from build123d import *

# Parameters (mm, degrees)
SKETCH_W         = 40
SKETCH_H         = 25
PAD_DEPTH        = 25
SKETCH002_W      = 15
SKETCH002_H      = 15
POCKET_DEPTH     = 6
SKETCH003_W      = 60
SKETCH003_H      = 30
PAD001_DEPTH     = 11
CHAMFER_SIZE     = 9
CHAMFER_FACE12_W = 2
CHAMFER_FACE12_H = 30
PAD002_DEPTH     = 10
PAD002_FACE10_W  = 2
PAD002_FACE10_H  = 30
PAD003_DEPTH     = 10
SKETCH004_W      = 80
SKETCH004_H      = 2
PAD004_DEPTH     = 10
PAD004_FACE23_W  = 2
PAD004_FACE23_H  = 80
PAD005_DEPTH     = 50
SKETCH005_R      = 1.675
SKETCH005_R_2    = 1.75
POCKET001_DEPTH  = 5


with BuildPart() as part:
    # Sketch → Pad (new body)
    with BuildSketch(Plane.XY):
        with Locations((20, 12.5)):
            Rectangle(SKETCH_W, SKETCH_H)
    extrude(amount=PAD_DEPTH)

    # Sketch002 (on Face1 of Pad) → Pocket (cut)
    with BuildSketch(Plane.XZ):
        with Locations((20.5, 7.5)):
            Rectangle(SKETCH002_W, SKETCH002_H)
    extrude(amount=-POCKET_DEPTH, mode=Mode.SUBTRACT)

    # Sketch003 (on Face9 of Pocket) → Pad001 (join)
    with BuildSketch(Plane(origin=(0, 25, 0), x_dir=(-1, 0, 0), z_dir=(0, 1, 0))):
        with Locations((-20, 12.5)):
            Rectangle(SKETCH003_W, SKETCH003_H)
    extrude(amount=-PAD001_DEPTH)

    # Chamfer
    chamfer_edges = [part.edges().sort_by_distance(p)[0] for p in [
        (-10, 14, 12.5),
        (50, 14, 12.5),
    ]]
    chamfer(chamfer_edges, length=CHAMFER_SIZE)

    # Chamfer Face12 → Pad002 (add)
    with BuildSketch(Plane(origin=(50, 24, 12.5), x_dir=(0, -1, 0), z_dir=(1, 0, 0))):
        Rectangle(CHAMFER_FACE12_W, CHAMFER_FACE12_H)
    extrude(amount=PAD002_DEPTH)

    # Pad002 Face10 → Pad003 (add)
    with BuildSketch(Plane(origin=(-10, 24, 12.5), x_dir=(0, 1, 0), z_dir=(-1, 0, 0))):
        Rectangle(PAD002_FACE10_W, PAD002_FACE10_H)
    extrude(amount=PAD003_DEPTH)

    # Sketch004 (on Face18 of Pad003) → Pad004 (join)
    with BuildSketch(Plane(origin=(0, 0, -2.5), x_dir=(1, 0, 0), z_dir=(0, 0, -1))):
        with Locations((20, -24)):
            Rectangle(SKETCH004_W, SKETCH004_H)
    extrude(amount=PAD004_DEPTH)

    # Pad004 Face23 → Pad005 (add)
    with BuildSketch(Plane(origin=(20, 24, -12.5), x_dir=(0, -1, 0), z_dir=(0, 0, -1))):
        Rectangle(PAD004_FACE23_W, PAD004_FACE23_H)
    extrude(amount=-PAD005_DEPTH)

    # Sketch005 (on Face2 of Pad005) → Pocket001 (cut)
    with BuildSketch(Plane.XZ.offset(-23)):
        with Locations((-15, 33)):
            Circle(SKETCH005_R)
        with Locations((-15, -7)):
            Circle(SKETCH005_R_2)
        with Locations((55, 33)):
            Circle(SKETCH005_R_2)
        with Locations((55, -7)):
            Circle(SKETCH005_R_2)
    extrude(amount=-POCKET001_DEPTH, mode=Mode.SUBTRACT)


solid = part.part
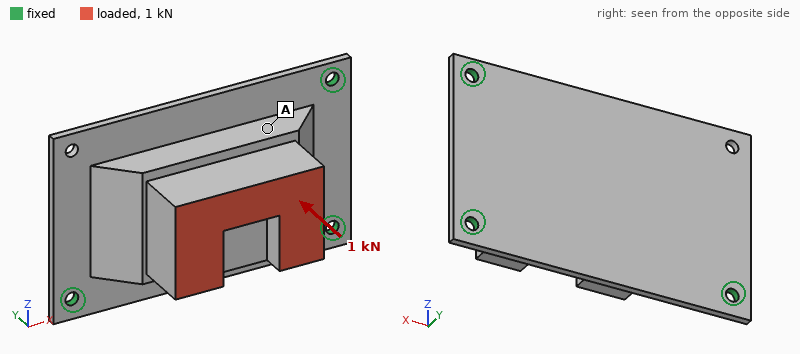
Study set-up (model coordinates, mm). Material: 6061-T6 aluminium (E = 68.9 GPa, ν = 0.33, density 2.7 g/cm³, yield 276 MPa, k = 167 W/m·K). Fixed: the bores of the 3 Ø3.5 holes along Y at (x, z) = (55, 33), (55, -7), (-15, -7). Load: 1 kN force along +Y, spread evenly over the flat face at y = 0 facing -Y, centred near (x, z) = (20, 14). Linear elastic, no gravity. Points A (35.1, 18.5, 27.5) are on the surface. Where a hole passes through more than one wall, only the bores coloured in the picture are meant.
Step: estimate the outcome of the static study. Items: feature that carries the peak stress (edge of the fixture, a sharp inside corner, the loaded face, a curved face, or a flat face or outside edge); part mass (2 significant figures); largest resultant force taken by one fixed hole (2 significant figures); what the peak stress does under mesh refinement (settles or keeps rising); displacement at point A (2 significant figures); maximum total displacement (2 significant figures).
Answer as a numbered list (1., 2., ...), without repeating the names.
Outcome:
1. edge of the fixture
2. 93 g
3. 690 N
4. keeps rising
5. 0.093 mm
6. 0.18 mm
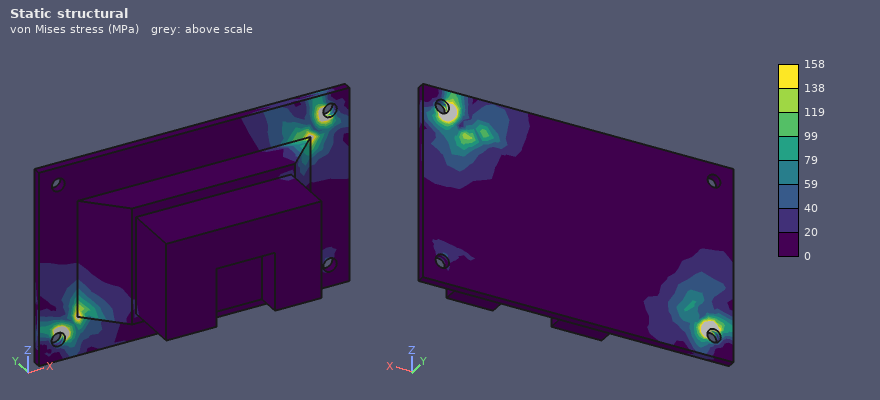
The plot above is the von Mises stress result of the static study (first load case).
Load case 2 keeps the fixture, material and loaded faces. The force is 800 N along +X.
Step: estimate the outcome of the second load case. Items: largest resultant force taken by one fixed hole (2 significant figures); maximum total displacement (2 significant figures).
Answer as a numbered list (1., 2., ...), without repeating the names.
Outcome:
1. 500 N
2. 99 µm
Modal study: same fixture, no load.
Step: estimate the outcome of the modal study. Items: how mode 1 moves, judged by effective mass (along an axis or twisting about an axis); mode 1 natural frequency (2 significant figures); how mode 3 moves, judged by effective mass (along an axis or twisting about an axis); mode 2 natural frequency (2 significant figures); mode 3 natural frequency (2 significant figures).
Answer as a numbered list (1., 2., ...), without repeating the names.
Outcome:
1. along Y
2. 1600 Hz
3. along X
4. 3200 Hz
5. 4400 Hz
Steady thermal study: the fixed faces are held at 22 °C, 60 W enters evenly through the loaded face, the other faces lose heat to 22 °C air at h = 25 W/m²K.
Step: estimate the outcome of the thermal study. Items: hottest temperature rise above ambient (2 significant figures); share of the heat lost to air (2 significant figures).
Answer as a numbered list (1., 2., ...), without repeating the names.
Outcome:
1. 50 K
2. 16 %
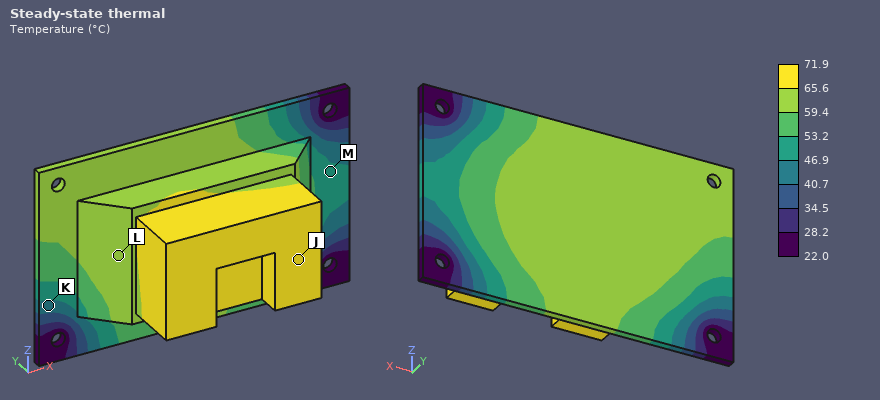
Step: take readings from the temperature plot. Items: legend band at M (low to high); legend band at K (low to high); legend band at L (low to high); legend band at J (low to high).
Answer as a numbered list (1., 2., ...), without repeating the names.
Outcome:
1. 46.9 to 53.2 °C
2. 40.7 to 46.9 °C
3. 59.4 to 65.6 °C
4. 65.6 to 71.9 °C
